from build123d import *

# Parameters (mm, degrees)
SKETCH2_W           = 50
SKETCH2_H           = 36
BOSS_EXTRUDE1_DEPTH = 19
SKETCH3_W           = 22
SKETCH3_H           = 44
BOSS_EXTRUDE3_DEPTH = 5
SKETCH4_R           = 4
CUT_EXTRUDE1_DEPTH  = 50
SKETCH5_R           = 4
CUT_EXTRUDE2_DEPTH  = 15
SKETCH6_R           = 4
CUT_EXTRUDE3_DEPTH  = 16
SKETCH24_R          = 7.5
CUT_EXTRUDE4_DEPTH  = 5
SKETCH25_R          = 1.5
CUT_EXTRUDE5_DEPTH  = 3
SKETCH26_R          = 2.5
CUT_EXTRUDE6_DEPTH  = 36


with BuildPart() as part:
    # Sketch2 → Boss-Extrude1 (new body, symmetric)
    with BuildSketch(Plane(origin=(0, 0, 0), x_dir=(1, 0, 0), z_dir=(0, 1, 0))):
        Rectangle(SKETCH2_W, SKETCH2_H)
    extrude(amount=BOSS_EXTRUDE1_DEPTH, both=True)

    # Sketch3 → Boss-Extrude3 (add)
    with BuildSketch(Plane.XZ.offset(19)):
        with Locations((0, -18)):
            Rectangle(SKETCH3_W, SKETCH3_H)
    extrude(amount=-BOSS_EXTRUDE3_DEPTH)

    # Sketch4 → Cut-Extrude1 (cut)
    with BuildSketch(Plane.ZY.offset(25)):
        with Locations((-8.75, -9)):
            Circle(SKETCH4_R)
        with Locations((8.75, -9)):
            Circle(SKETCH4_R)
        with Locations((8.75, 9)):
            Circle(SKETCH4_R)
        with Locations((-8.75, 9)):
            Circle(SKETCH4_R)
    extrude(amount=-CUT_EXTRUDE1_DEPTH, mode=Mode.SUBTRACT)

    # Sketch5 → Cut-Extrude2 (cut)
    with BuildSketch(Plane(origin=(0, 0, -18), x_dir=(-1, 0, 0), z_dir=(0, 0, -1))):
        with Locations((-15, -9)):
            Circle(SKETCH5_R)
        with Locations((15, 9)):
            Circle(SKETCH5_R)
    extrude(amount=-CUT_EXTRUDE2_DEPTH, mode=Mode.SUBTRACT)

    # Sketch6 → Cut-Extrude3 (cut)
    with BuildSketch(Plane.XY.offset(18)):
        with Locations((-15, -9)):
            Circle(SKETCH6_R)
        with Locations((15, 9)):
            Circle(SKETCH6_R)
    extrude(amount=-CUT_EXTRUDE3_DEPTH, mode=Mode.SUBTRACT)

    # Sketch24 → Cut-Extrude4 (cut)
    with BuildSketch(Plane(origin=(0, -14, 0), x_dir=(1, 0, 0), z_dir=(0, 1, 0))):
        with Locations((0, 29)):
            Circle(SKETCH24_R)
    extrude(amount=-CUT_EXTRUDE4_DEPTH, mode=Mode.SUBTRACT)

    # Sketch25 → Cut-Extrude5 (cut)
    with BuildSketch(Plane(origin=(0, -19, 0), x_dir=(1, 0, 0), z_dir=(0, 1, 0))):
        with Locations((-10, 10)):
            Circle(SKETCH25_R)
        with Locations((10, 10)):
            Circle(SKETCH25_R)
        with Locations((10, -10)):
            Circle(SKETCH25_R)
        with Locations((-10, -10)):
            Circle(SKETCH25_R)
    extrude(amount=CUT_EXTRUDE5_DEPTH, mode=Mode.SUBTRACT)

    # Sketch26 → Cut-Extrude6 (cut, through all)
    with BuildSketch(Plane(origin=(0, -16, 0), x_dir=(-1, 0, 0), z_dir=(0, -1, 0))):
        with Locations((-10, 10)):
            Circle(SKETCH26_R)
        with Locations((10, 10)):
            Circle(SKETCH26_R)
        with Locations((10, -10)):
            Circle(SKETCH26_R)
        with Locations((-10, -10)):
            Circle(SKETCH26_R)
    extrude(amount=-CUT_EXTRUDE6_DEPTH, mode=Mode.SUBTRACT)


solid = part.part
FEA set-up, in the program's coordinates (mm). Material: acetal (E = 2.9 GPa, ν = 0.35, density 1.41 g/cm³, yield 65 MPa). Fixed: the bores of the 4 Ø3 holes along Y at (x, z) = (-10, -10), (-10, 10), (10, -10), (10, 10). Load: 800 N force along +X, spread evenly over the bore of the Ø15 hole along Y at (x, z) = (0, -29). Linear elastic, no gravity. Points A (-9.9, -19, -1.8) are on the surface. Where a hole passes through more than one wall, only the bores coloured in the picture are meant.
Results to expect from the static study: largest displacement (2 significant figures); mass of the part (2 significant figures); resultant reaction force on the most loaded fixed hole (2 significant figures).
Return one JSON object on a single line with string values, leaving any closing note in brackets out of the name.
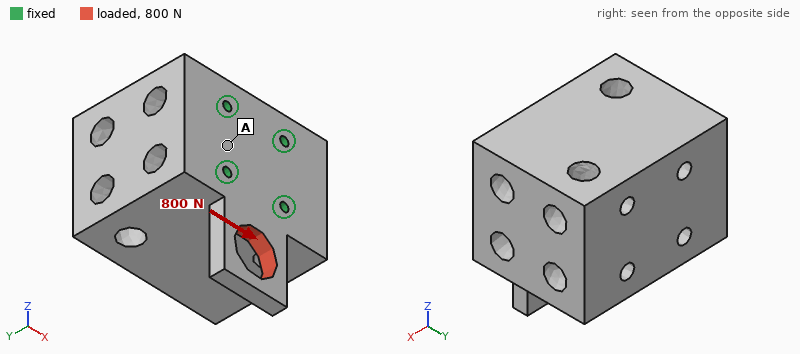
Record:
{"largest displacement": "0.92 mm", "mass of the part": "80 g", "resultant reaction force on the most loaded fixed hole": "660 N"}
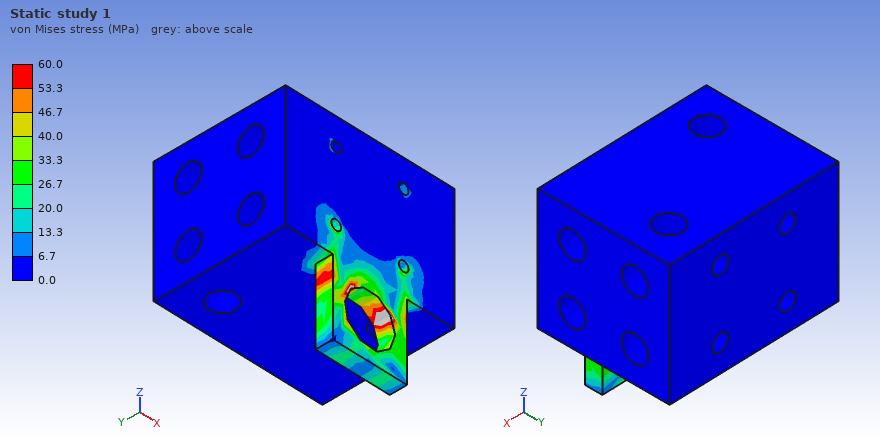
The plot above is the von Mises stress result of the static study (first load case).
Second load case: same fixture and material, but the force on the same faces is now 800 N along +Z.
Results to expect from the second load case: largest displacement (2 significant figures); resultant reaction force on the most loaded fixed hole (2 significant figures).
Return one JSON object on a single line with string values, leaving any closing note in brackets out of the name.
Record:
{"largest displacement": "0.20 mm", "resultant reaction force on the most loaded fixed hole": "310 N"}
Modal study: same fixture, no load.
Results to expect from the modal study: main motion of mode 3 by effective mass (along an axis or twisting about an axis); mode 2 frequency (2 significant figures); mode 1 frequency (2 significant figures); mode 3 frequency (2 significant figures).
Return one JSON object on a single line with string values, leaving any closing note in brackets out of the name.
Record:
{"main motion of mode 3 by effective mass": "along Z", "mode 2 frequency": "1400 Hz", "mode 1 frequency": "1400 Hz", "mode 3 frequency": "1800 Hz"}
